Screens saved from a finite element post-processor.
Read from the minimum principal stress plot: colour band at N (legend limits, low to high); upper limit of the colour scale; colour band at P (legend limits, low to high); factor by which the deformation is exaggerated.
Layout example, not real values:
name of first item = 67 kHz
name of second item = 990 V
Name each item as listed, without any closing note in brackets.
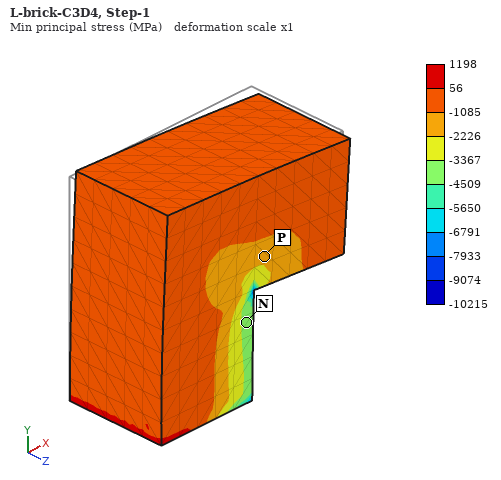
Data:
colour band at N = -4509 to -3367 MPa
upper limit of the colour scale = 1198 MPa
colour band at P = -2226 to -1085 MPa
factor by which the deformation is exaggerated = 1
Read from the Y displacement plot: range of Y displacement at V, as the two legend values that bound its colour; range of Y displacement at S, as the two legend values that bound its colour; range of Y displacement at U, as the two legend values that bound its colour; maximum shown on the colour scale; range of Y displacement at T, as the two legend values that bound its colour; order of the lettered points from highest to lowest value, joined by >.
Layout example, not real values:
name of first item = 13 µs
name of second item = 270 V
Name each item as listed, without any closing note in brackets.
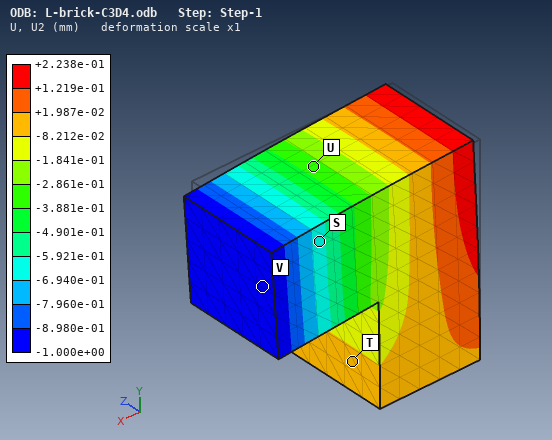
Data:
range of Y displacement at V, as the two legend values that bound its colour = -1.000e+00 to -8.980e-01 mm
range of Y displacement at S, as the two legend values that bound its colour = -6.940e-01 to -5.921e-01 mm
range of Y displacement at U, as the two legend values that bound its colour = -3.881e-01 to -2.861e-01 mm
maximum shown on the colour scale = +2.238e-01 mm
range of Y displacement at T, as the two legend values that bound its colour = -8.212e-02 to +1.987e-02 mm
order of the lettered points from highest to lowest value, joined by > = T > U > S > V
